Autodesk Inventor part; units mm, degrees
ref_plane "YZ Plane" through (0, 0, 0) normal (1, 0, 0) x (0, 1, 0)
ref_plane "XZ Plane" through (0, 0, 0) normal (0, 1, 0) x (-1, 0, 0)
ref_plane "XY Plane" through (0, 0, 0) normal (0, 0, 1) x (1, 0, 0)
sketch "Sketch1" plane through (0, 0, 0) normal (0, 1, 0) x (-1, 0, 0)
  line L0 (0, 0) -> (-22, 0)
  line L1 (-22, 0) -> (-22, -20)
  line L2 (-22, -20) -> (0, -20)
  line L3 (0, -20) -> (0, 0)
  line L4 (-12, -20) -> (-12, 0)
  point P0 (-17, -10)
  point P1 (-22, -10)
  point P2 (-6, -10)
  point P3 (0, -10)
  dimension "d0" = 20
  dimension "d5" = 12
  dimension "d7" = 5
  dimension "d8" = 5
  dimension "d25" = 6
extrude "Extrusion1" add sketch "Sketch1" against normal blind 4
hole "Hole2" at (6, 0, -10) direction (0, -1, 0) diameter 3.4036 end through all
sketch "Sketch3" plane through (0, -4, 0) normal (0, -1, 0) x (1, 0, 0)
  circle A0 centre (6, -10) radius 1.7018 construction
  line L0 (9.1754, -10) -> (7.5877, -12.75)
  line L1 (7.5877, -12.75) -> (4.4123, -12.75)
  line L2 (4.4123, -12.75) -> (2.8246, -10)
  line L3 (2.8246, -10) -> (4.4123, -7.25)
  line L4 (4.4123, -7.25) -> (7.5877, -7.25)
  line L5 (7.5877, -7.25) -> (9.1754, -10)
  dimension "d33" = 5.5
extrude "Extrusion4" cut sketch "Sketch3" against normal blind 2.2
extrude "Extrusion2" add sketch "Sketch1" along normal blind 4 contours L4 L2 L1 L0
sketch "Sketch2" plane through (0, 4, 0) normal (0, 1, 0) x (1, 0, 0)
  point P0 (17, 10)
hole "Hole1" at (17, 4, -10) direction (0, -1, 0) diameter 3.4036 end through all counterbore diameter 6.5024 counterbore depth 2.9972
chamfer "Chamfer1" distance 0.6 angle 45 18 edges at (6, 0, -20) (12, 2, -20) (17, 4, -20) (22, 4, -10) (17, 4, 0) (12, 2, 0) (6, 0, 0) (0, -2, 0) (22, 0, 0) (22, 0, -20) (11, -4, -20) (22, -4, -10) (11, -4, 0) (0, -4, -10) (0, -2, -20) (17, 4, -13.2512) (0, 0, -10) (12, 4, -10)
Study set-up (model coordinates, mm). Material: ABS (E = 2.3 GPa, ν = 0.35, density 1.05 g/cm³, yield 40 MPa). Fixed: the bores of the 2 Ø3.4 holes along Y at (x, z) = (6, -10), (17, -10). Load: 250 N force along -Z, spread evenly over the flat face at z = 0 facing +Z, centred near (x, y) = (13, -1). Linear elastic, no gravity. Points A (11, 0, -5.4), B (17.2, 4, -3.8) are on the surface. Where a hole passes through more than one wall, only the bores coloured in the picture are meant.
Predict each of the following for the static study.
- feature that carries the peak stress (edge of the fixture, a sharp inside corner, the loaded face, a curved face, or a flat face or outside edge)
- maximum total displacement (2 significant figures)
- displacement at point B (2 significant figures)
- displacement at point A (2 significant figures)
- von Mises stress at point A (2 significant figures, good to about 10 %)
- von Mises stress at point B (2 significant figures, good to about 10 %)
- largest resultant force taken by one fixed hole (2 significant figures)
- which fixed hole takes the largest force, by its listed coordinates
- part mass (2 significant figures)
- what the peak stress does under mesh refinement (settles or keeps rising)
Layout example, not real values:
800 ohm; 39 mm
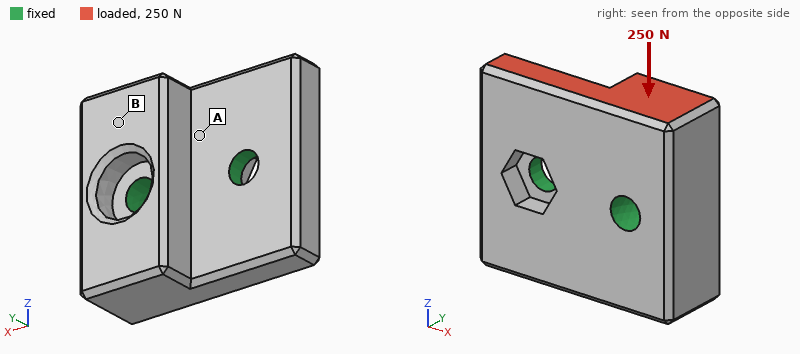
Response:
edge of the fixture; 23 µm; 18 µm; 8.0 µm; 2.2 MPa; 1.1 MPa; 170 N; (17, -10); 2.4 g; keeps rising
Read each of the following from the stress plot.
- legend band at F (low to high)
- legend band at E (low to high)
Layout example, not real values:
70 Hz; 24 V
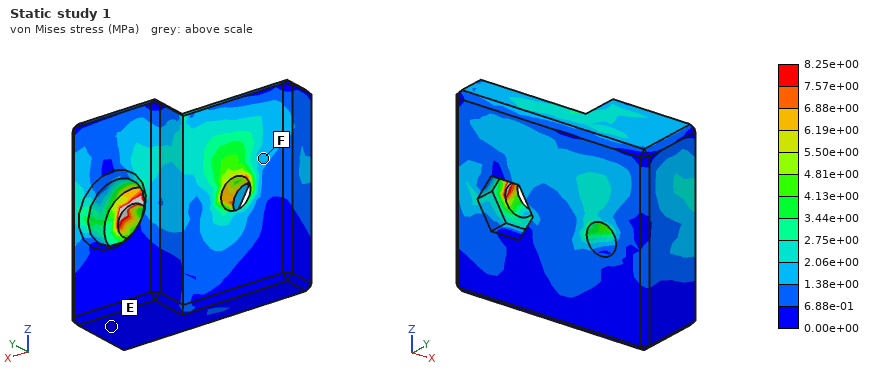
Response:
1.38e+00 to 2.06e+00 MPa; 0.00e+00 to 6.88e-01 MPa
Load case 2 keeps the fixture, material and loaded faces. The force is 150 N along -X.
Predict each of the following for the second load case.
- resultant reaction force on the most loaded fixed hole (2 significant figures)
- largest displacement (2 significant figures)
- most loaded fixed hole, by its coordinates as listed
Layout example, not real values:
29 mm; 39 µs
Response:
140 N; 46 µm; (17, -10)
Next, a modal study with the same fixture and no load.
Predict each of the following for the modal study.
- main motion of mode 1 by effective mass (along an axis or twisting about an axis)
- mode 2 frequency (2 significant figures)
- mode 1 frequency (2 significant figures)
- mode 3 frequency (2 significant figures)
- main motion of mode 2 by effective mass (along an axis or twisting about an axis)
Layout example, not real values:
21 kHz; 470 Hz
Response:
twisting about X; 9400 Hz; 6700 Hz; 10000 Hz; along Y
